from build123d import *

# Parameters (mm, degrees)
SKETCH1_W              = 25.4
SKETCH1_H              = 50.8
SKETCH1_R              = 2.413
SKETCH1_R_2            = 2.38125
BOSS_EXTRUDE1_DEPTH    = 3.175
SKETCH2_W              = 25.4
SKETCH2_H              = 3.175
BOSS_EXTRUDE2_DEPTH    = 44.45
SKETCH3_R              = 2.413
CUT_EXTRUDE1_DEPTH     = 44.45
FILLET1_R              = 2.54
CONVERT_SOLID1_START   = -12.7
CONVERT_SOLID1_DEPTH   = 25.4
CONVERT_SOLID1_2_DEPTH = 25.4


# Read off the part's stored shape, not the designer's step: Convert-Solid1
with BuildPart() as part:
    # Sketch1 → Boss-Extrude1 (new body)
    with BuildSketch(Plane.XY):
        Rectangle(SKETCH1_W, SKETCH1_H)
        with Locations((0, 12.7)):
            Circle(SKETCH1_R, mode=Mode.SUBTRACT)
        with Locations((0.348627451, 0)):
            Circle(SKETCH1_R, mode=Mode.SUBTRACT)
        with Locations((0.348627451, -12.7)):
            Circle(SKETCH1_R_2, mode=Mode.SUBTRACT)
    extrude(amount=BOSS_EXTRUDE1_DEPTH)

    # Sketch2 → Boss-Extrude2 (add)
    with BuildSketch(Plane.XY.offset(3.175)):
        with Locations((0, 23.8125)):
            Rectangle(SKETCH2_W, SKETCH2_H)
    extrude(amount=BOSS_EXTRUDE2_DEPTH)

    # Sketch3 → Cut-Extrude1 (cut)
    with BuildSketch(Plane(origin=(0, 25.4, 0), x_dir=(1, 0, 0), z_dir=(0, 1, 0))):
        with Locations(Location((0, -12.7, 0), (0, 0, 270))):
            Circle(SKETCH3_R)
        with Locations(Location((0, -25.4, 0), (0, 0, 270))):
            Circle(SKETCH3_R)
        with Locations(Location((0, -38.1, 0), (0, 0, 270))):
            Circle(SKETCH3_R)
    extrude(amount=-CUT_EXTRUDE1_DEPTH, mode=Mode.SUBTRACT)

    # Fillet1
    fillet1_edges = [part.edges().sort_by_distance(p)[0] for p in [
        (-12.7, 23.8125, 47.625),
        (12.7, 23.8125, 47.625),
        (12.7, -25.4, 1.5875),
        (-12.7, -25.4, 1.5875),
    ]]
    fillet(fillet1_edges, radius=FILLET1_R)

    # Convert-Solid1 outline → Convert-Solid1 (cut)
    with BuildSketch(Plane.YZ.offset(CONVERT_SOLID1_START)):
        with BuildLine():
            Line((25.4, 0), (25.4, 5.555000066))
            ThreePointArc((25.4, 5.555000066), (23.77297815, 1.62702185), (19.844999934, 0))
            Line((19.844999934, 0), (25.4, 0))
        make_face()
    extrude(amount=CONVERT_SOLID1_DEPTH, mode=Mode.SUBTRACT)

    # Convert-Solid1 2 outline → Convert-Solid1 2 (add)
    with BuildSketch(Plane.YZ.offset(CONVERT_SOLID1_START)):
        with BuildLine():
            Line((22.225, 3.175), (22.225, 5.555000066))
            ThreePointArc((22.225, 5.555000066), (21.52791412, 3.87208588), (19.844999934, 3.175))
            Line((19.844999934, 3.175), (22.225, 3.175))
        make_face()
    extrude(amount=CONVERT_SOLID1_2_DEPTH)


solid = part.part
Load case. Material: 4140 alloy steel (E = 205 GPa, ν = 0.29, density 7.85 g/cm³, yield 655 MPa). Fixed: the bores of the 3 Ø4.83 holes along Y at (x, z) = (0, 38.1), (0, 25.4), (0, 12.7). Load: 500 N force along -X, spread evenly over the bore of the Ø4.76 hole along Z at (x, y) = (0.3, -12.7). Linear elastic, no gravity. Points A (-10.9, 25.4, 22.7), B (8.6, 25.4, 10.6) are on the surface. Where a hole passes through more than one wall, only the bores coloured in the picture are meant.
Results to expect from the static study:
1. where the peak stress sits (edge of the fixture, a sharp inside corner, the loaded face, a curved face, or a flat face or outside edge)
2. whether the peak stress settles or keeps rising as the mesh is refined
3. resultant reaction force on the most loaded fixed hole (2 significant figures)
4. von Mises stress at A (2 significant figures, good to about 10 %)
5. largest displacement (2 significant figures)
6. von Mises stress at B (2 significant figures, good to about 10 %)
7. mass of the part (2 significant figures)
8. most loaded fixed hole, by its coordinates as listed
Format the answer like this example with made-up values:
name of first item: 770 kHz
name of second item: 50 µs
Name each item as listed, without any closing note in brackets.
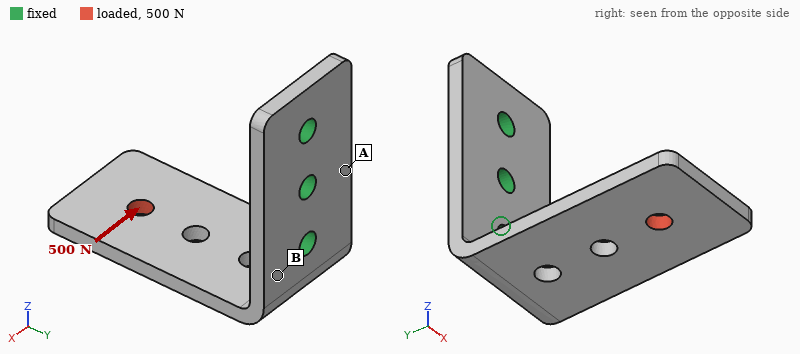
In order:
where the peak stress sits: edge of the fixture
whether the peak stress settles or keeps rising as the mesh is refined: keeps rising
resultant reaction force on the most loaded fixed hole: 680 N
von Mises stress at A: 74 MPa
largest displacement: 0.38 mm
von Mises stress at B: 180 MPa
mass of the part: 56 g
most loaded fixed hole, by its coordinates as listed: (0, 12.7)
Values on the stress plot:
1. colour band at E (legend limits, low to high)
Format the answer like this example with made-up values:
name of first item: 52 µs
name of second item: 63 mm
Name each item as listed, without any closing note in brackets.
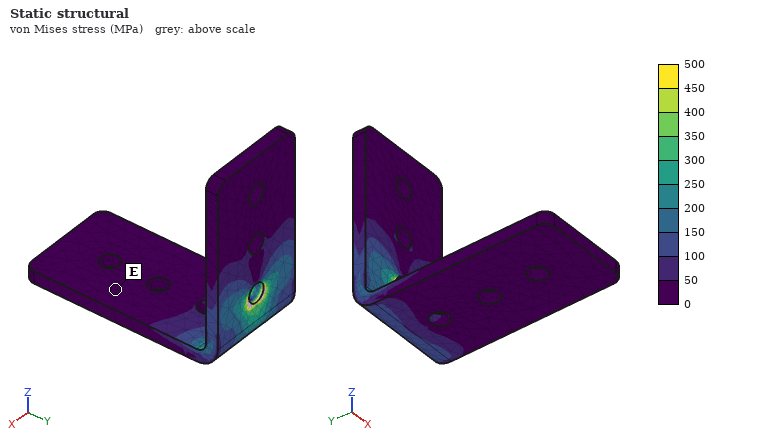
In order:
colour band at E: 0 to 50 MPa
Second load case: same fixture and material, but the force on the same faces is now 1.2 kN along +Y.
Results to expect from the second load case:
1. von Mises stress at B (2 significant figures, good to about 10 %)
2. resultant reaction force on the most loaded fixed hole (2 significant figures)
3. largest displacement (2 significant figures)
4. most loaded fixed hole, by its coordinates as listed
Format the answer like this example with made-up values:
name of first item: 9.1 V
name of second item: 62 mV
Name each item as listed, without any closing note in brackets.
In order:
von Mises stress at B: 130 MPa
resultant reaction force on the most loaded fixed hole: 1.5 kN
largest displacement: 0.25 mm
most loaded fixed hole, by its coordinates as listed: (0, 12.7)
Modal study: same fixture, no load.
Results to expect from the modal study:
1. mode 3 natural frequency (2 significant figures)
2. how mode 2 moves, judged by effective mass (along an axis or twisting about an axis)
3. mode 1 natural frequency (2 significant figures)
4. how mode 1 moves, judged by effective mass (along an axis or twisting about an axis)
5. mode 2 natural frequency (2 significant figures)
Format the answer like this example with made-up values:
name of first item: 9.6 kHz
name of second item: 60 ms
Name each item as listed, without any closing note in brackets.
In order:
mode 3 natural frequency: 4100 Hz
how mode 2 moves, judged by effective mass: along X
mode 1 natural frequency: 830 Hz
how mode 1 moves, judged by effective mass: along Z
mode 2 natural frequency: 1500 Hz
